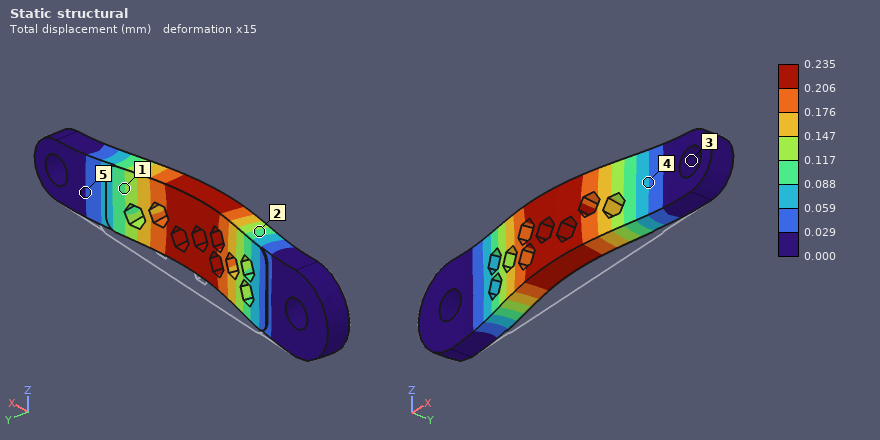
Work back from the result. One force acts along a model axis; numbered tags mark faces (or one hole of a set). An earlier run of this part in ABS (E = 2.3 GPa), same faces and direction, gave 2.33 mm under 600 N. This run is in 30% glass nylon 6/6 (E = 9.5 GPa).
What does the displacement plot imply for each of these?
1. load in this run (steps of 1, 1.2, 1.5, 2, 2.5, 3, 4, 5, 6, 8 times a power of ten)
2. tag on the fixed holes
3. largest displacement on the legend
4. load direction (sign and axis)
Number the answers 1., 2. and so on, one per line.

1. 250 N
2. 3
3. 0.235 mm
4. -Y
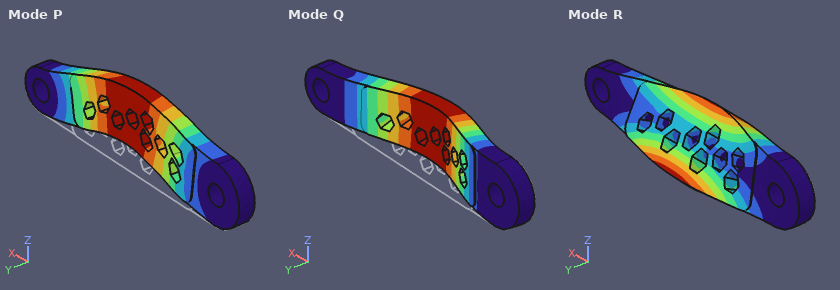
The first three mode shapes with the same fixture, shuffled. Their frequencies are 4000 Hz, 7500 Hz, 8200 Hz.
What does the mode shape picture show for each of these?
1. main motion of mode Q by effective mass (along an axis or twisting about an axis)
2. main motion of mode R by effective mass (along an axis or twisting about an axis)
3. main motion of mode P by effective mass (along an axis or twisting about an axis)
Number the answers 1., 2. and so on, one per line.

1. along Y
2. twisting about X
3. along Z
